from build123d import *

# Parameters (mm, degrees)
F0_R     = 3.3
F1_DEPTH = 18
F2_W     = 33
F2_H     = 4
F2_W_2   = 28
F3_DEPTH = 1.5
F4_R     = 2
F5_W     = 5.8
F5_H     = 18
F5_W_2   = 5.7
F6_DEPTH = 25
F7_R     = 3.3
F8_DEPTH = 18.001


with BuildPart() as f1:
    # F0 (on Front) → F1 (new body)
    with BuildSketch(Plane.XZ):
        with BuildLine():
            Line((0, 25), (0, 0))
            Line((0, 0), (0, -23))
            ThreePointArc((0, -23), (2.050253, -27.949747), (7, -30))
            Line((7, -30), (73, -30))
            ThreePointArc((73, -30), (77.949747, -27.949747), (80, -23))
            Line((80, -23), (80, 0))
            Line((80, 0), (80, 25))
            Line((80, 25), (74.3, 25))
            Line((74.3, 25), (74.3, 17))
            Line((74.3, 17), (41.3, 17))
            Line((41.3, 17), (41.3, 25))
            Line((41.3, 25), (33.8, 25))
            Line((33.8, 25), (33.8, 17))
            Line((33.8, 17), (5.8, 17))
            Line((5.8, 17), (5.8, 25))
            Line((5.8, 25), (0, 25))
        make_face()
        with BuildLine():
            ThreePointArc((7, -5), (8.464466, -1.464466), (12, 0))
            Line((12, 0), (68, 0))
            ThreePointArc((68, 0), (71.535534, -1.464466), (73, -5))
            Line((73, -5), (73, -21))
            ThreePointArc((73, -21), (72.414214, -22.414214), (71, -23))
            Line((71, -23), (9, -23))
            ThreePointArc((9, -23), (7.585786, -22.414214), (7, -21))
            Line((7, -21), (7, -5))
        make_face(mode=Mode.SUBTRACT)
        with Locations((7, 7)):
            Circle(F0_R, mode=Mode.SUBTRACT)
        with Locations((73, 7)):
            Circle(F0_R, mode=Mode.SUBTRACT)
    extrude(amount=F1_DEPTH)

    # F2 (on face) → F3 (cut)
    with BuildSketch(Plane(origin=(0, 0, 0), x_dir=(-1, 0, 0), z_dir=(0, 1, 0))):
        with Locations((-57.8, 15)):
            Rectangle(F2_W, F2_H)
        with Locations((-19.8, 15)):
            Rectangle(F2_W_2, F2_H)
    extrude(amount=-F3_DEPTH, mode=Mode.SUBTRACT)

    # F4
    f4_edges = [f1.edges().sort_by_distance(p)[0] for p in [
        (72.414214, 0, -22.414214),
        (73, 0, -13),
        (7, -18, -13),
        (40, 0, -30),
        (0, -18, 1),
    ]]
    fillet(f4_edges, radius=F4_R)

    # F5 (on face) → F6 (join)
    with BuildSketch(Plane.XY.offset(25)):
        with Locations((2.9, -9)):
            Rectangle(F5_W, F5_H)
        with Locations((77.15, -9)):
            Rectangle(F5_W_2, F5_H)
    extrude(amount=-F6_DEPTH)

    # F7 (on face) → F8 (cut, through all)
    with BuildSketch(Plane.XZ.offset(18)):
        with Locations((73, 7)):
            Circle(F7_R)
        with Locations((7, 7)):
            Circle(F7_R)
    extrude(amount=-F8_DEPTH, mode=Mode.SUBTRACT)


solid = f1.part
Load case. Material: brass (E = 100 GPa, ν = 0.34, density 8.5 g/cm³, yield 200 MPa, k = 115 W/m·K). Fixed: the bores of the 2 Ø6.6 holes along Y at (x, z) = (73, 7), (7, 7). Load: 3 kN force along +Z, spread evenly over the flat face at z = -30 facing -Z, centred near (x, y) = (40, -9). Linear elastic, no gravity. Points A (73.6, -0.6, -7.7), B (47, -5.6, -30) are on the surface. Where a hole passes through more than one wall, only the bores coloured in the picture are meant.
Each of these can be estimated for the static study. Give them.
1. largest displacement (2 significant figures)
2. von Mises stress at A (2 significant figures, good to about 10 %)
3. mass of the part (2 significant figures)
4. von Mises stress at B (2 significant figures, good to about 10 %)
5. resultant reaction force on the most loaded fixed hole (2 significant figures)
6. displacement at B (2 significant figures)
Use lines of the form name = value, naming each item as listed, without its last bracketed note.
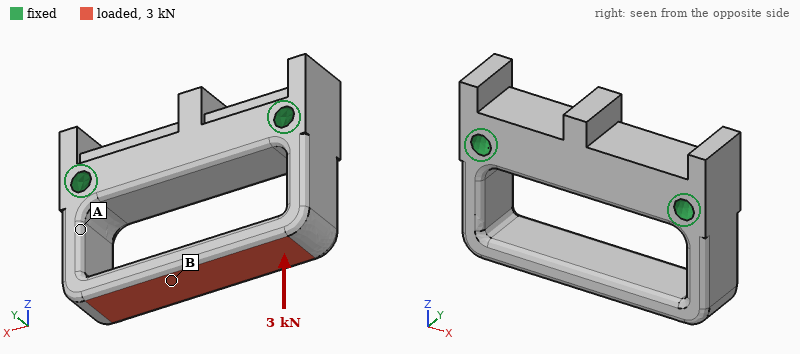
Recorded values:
largest displacement = 0.11 mm
von Mises stress at A = 24 MPa
mass of the part = 350 g
von Mises stress at B = 84 MPa
resultant reaction force on the most loaded fixed hole = 1.7 kN
displacement at B = 0.100 mm
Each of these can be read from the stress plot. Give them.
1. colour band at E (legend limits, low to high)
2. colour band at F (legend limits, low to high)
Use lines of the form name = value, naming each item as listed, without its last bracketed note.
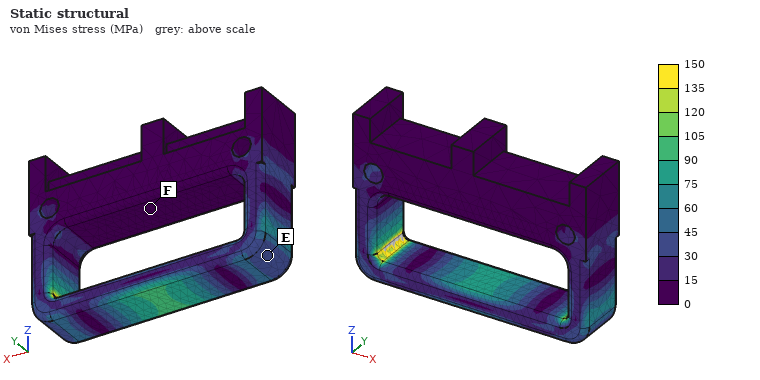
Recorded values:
colour band at E = 30 to 45 MPa
colour band at F = 0 to 15 MPa
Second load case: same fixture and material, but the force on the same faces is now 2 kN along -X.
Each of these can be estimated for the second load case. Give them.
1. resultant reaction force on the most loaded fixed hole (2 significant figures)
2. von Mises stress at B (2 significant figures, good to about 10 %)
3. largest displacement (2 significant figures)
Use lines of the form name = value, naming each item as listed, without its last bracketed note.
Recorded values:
resultant reaction force on the most loaded fixed hole = 1.2 kN
von Mises stress at B = 13 MPa
largest displacement = 75 µm
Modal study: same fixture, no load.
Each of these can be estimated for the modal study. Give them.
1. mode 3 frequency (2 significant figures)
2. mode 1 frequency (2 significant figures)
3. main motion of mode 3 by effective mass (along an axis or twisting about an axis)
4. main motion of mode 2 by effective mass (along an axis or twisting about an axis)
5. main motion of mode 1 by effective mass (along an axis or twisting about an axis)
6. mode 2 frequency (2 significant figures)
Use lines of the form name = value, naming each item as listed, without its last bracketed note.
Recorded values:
mode 3 frequency = 3600 Hz
mode 1 frequency = 2800 Hz
main motion of mode 3 by effective mass = along Z
main motion of mode 2 by effective mass = along Y
main motion of mode 1 by effective mass = along X
mode 2 frequency = 3200 Hz
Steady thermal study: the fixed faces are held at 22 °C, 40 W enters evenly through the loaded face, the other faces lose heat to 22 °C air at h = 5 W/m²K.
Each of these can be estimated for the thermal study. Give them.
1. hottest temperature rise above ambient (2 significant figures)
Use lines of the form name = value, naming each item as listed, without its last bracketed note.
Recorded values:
hottest temperature rise above ambient = 65 K
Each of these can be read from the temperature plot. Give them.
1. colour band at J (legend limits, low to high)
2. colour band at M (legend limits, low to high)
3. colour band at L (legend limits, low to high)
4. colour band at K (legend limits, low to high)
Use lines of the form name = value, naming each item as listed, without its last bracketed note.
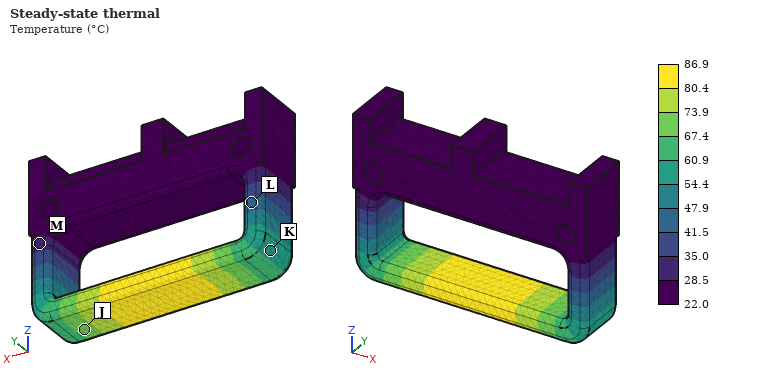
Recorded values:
colour band at J = 67.4 to 73.9 °C
colour band at M = 28.5 to 35.0 °C
colour band at L = 41.5 to 47.9 °C
colour band at K = 54.4 to 60.9 °C
